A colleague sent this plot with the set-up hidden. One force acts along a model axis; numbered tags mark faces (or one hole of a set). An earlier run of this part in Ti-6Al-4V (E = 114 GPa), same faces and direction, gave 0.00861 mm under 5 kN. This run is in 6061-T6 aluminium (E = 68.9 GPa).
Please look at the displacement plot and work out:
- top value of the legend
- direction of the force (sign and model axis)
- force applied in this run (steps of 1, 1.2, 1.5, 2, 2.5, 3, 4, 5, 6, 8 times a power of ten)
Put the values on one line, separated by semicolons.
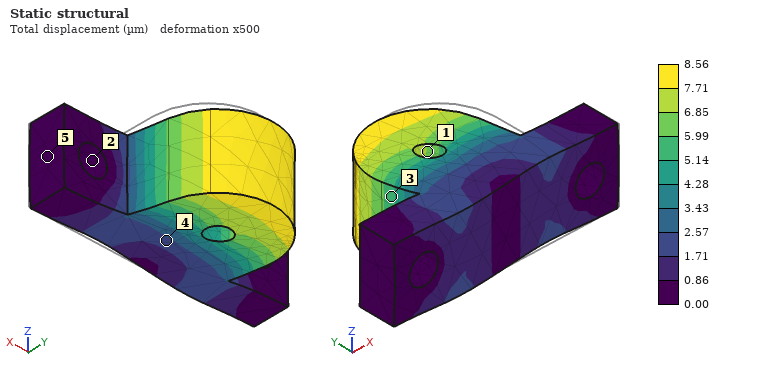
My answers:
8.56 µm; -X; 3 kN
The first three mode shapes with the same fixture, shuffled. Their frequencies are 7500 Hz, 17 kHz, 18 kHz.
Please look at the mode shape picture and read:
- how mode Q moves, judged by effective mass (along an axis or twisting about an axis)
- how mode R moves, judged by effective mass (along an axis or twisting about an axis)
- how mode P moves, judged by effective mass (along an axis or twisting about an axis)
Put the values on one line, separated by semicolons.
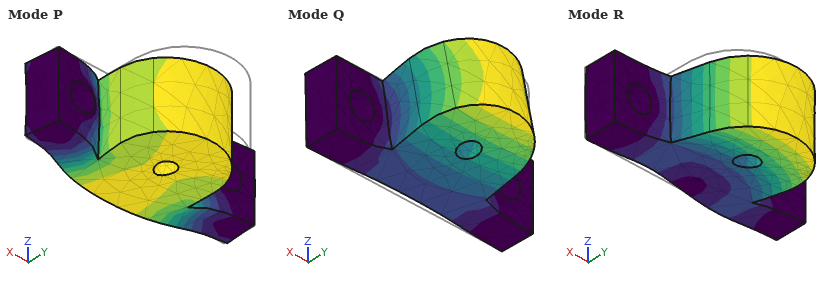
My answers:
along Z; along X; along Y
